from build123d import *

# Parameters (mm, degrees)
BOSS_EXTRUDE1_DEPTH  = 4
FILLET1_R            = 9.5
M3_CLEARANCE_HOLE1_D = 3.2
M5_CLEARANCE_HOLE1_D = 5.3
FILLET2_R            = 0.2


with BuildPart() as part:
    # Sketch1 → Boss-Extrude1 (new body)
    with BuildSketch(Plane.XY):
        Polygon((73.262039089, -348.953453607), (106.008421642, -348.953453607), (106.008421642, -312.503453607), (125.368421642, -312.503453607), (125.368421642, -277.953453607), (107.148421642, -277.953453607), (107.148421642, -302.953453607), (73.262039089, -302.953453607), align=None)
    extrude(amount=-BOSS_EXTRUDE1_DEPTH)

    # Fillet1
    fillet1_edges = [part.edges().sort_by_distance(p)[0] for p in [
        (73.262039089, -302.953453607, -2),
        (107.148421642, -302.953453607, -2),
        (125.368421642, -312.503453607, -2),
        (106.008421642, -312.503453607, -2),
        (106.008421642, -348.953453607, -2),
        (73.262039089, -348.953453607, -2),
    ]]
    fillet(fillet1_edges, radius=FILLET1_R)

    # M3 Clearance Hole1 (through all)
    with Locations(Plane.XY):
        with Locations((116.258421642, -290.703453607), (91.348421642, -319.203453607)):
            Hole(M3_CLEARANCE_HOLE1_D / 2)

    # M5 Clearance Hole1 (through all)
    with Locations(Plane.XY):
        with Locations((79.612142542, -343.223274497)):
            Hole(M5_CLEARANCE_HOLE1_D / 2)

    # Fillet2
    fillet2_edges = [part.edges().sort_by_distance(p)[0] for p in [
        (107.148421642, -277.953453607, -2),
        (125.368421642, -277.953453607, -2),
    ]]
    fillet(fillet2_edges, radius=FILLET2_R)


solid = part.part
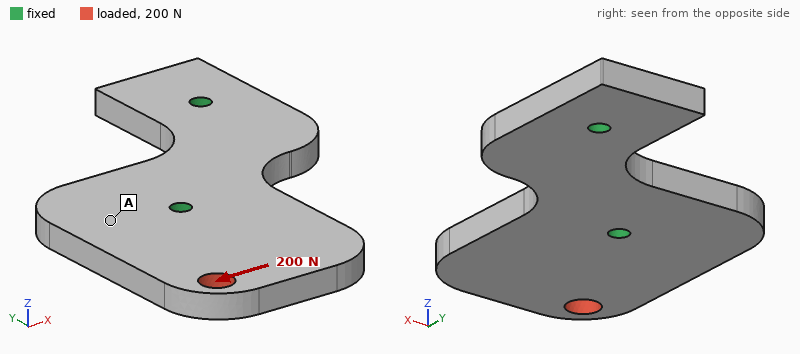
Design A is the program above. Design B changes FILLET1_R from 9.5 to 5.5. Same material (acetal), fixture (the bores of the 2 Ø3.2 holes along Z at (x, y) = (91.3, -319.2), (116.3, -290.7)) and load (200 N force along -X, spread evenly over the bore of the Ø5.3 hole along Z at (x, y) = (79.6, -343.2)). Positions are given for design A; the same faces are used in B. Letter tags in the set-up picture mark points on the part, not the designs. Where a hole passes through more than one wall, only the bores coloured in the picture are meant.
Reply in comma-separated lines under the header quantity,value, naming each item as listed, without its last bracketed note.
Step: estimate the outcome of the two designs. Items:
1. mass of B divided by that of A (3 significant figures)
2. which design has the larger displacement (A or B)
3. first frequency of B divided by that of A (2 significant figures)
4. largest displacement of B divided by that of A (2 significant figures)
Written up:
quantity,value
mass of B divided by that of A,1.01
which design has the larger displacement,B
first frequency of B divided by that of A,0.95
largest displacement of B divided by that of A,1.2
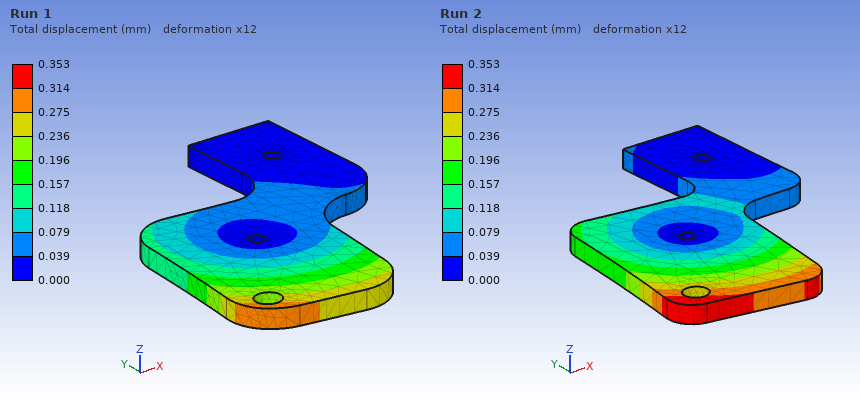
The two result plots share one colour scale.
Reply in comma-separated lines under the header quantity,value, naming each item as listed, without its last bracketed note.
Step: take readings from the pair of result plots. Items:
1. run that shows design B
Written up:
quantity,value
run that shows design B,Run 2
